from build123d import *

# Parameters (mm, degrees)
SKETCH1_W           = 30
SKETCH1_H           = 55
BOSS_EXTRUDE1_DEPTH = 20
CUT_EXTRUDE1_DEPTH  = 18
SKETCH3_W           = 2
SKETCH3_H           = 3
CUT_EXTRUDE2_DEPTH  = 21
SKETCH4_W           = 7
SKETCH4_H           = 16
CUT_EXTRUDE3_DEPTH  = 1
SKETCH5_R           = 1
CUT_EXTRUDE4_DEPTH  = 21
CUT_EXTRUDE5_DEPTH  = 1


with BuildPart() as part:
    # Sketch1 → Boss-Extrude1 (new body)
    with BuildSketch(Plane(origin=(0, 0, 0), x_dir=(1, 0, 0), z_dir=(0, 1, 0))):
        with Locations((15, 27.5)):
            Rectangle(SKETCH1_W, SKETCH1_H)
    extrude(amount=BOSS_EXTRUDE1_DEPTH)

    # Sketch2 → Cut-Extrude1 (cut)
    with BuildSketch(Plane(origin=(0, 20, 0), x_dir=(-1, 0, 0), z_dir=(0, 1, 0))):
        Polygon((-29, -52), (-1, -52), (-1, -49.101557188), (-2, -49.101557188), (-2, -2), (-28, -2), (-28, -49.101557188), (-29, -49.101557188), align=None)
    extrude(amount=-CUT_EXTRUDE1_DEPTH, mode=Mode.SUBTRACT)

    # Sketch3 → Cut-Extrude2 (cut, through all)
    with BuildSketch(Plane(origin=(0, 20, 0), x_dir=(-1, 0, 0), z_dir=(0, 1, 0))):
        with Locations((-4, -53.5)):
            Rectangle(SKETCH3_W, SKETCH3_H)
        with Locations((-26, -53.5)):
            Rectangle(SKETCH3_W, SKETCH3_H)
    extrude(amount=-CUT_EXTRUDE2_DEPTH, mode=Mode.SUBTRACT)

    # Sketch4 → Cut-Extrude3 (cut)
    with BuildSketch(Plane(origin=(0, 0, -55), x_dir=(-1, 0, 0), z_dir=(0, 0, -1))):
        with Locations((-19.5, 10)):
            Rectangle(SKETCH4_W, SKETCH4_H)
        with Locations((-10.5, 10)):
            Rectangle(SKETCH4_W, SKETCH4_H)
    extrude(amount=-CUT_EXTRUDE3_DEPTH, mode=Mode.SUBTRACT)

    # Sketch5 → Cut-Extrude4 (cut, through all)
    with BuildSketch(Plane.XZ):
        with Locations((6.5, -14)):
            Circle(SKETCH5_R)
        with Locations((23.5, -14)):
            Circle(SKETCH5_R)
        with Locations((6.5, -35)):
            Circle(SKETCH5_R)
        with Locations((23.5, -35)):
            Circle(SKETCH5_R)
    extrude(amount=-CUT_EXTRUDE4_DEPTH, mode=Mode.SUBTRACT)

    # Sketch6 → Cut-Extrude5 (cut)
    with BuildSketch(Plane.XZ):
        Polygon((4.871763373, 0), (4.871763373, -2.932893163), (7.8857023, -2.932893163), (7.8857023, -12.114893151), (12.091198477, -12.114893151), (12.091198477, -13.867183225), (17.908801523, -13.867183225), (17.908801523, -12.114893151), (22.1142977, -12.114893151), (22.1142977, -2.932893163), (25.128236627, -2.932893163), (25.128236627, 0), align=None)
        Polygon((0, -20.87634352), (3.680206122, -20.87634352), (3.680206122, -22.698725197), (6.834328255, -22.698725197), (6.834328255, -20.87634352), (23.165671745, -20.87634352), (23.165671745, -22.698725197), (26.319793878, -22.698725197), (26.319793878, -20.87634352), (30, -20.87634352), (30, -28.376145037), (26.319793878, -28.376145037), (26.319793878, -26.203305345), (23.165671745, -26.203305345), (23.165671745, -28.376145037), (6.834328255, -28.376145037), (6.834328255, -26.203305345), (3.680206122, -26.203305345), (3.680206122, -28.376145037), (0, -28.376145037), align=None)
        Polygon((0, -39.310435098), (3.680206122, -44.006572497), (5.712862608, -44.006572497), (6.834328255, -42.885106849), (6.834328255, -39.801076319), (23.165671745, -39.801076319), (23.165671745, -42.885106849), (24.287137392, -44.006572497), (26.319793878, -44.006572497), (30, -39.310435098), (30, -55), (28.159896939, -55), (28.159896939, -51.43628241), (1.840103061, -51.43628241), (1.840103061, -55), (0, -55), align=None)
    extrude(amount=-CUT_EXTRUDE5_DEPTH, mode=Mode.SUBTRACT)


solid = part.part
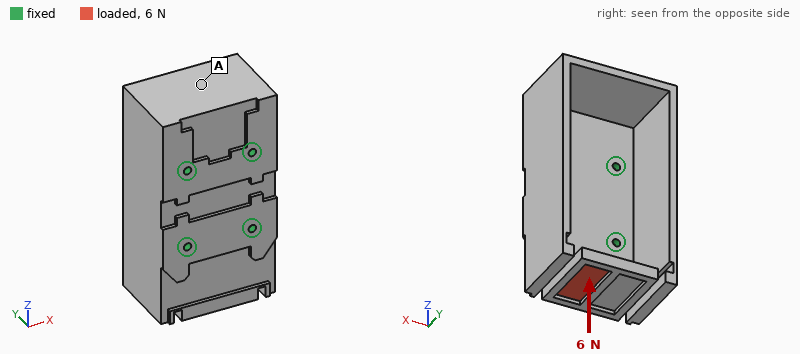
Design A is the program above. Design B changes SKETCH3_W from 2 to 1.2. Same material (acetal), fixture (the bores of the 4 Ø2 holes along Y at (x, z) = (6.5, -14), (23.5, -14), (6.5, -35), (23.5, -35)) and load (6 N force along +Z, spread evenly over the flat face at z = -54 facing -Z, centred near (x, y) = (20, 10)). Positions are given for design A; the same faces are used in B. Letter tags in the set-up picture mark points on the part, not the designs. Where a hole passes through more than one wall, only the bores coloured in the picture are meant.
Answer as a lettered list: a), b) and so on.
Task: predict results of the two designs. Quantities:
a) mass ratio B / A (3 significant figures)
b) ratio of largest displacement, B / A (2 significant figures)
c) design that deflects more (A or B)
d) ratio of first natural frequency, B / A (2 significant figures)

a) 1.01
b) 0.88
c) A
d) 1.0
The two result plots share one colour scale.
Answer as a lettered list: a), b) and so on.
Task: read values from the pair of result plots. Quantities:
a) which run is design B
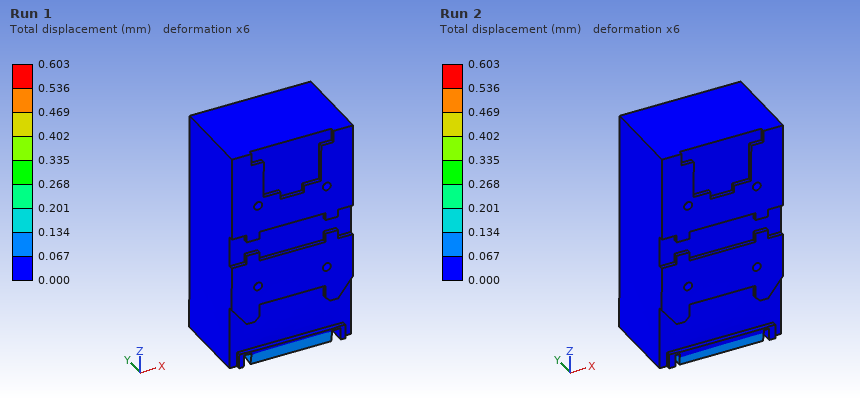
a) Run 2
